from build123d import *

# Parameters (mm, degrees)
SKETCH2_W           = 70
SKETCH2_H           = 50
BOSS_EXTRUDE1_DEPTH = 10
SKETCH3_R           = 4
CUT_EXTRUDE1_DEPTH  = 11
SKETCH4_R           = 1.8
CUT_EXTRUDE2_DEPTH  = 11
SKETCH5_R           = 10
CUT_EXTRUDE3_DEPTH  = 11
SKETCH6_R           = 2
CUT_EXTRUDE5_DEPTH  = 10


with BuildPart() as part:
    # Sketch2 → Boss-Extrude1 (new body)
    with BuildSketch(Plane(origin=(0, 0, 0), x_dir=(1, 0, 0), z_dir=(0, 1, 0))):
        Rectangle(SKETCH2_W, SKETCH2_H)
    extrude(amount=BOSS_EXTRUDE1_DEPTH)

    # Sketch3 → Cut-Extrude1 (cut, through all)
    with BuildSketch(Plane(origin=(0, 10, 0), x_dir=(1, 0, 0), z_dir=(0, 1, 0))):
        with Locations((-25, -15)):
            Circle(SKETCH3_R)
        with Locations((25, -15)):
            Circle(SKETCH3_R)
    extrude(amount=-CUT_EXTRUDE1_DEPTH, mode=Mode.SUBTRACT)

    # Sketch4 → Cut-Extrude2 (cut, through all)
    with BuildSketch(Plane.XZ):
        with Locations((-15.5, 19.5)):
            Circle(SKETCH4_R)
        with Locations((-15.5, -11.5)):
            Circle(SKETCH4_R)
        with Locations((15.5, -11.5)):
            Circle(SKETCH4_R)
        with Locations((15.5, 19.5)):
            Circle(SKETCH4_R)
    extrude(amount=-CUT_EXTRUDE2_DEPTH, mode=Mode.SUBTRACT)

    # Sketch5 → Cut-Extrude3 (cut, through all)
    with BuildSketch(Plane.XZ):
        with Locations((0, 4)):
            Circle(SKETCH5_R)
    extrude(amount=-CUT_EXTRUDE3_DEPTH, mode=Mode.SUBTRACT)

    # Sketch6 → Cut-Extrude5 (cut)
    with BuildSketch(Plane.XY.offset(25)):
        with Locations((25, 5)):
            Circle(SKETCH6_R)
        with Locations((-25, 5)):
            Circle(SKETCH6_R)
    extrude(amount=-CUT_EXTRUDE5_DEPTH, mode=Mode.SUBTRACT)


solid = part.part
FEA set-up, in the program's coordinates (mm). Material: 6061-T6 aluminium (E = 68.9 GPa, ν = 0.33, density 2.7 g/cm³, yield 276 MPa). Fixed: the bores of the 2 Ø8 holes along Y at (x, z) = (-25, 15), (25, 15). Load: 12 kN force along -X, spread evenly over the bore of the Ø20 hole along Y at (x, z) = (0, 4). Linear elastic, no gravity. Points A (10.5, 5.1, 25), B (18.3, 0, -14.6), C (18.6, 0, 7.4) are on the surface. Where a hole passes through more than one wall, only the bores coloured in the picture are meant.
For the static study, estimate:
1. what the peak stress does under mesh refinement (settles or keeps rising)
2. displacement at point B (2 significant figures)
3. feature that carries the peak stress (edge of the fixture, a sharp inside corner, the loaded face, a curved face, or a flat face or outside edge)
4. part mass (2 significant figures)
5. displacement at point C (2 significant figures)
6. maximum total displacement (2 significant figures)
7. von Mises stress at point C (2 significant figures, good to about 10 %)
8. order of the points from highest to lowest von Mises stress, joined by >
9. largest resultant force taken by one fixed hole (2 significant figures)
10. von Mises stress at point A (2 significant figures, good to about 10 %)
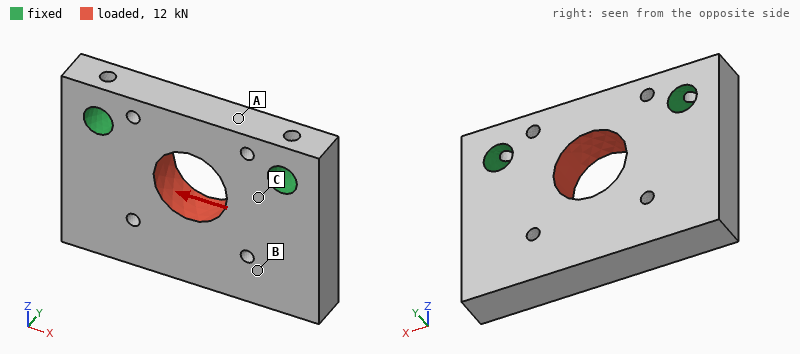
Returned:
keeps rising
18 µm
edge of the fixture
82 g
6.4 µm
21 µm
35 MPa
C > A > B
6.3 kN
18 MPa
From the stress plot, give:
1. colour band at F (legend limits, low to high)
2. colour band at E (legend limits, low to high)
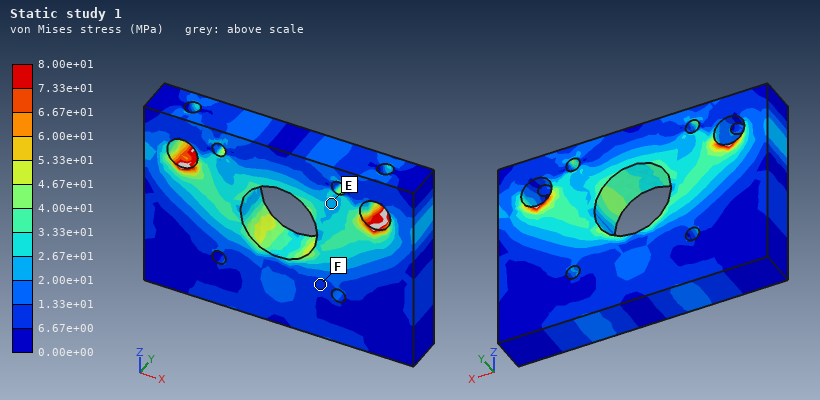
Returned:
6.67e+00 to 1.33e+01 MPa
2.00e+01 to 2.67e+01 MPa
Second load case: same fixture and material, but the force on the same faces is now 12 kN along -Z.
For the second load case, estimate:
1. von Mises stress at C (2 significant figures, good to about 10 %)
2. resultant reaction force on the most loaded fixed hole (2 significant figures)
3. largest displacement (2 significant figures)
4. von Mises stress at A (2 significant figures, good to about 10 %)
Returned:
39 MPa
6.1 kN
20 µm
17 MPa
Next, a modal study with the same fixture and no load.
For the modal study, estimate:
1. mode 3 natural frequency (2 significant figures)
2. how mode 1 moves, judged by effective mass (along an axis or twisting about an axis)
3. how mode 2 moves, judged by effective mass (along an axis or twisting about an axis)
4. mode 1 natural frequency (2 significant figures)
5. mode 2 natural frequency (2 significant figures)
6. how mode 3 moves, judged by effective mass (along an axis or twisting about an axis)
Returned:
13 kHz
along Y
twisting about Z
4400 Hz
7600 Hz
along X
